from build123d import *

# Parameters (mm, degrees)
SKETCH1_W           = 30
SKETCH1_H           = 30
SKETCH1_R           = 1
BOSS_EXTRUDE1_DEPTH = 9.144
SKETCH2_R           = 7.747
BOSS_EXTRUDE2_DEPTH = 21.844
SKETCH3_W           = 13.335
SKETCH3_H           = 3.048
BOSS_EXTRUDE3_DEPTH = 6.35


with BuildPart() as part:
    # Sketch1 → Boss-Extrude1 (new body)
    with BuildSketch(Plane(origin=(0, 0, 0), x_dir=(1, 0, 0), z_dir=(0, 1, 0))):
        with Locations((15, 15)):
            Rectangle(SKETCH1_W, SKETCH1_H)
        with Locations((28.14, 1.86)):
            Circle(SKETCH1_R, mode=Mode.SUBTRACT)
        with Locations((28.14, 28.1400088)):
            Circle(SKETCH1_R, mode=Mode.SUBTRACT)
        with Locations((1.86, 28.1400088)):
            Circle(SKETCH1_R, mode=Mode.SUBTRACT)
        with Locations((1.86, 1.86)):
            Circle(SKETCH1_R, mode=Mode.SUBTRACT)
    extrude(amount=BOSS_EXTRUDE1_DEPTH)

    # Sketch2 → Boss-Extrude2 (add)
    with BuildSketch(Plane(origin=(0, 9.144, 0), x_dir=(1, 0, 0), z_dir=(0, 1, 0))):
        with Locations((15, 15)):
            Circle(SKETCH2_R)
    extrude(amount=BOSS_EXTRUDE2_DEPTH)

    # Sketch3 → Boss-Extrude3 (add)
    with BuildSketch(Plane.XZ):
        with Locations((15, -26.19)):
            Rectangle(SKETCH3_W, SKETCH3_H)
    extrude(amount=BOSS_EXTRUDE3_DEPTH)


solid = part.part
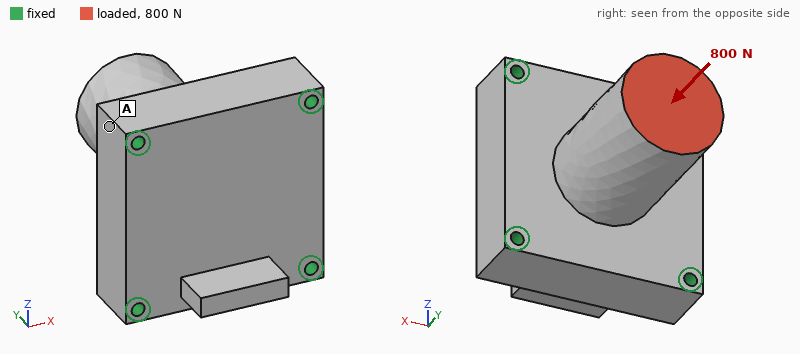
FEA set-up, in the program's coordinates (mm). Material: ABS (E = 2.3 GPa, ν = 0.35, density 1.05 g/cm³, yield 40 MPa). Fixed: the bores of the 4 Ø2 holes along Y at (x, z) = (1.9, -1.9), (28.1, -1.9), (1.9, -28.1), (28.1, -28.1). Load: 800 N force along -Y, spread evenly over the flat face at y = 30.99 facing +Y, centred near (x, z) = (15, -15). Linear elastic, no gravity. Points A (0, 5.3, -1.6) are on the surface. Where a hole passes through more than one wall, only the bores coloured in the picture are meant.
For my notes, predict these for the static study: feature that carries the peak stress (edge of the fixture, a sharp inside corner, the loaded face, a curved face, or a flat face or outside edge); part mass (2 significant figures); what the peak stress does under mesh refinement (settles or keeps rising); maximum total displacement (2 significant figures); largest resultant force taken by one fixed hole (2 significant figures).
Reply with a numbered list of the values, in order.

1. edge of the fixture
2. 13 g
3. keeps rising
4. 100 µm
5. 200 N
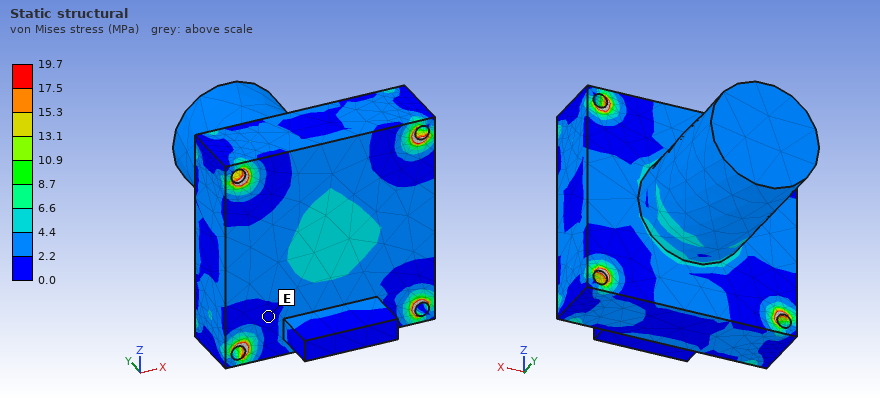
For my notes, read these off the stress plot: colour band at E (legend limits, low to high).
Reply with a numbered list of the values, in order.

1. 0.0 to 2.2 MPa
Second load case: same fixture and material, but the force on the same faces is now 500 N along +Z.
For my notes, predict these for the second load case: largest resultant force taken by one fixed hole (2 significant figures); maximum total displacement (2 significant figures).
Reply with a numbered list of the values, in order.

1. 310 N
2. 0.66 mm
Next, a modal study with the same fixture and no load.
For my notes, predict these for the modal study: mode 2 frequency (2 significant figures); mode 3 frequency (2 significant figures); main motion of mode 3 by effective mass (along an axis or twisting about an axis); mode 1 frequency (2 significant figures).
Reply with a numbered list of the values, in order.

1. 3700 Hz
2. 6000 Hz
3. along Y
4. 3700 Hz
